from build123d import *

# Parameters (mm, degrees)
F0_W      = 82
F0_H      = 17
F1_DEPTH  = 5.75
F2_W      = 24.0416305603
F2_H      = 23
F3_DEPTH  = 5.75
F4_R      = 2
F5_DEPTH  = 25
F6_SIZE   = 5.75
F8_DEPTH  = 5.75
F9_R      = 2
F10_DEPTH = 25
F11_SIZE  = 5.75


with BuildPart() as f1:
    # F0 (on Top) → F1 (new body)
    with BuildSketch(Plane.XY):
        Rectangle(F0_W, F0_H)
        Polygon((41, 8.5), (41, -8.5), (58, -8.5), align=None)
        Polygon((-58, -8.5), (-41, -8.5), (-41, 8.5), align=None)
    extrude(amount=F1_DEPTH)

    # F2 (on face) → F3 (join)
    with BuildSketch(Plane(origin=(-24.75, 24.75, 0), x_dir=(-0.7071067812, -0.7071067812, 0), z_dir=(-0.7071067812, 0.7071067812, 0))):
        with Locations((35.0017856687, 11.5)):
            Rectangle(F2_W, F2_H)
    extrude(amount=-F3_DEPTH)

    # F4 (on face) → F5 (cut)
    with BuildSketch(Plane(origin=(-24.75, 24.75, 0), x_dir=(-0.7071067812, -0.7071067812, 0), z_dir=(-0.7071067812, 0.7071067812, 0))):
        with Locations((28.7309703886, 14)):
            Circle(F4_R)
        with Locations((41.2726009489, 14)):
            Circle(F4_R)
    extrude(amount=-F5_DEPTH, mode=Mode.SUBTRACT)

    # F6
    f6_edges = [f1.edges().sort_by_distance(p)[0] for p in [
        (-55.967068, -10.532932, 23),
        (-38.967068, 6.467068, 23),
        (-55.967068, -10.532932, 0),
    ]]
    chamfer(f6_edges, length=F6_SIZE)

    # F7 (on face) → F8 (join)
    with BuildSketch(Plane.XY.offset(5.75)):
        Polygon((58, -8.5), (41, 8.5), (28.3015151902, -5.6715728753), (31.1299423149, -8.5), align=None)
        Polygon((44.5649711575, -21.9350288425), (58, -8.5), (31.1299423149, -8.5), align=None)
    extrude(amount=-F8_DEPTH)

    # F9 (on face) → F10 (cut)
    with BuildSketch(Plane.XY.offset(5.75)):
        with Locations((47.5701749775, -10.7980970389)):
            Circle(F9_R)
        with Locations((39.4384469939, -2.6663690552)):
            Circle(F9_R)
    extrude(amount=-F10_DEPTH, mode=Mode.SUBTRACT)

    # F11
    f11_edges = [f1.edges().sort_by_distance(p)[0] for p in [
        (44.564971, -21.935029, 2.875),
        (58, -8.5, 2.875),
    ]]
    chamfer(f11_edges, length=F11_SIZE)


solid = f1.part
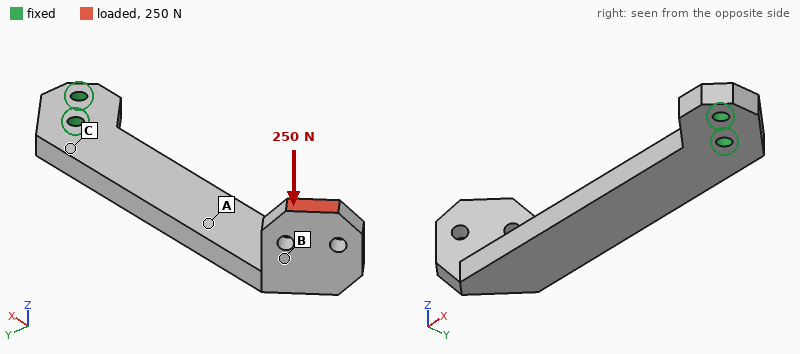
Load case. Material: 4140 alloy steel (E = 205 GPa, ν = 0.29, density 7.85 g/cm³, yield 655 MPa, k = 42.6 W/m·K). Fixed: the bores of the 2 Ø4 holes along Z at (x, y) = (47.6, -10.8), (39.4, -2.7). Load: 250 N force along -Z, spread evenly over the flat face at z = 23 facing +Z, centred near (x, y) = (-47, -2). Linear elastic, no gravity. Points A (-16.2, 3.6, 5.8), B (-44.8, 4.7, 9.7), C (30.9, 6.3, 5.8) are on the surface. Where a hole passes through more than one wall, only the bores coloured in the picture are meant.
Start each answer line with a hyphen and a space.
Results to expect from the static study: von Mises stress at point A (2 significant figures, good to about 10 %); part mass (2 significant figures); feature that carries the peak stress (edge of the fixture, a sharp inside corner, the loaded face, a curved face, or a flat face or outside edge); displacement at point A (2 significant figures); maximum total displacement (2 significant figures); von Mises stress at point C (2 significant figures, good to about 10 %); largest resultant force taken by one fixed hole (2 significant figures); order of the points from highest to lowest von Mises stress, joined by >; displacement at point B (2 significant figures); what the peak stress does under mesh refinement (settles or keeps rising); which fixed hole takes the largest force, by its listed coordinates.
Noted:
- 84 MPa
- 98 g
- edge of the fixture
- 0.47 mm
- 1.2 mm
- 180 MPa
- 700 N
- C > A > B
- 0.94 mm
- keeps rising
- (39.4, -2.7)
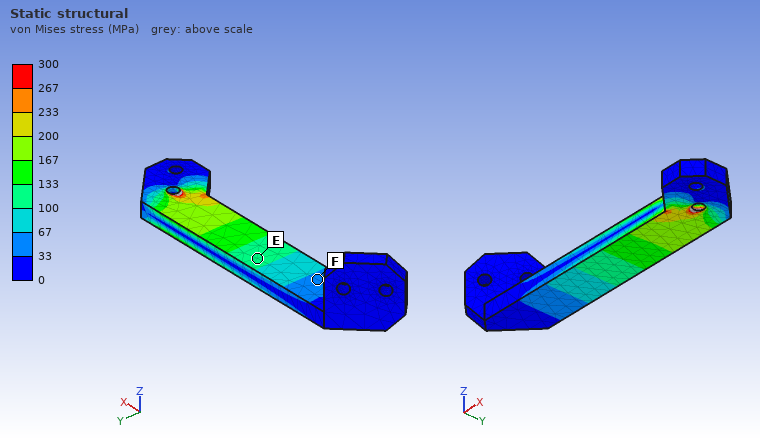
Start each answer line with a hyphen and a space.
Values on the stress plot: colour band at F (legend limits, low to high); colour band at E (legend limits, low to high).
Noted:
- 33 to 67 MPa
- 100 to 133 MPa
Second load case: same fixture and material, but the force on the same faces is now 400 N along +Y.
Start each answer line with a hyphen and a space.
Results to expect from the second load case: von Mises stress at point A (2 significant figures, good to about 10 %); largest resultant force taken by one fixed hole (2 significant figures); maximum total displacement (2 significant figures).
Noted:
- 99 MPa
- 2.2 kN
- 0.44 mm
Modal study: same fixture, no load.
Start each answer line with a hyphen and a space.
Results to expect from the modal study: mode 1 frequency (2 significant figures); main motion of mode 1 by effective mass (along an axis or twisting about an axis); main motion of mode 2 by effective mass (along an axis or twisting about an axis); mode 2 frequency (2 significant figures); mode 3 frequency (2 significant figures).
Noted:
- 430 Hz
- along Z
- along Y
- 1100 Hz
- 2600 Hz
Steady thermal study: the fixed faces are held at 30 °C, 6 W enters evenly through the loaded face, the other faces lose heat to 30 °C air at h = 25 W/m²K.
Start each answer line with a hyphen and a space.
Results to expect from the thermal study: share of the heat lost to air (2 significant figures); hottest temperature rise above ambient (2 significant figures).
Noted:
- 68 %
- 75 K
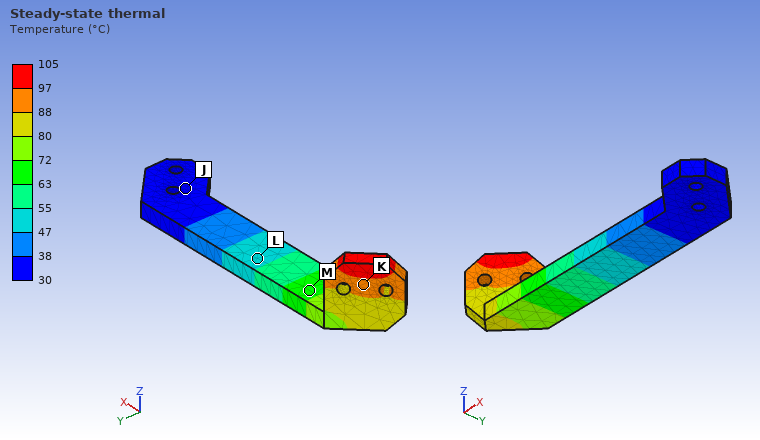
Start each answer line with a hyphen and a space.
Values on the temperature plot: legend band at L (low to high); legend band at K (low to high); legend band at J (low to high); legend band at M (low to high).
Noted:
- 47 to 55 °C
- 88 to 97 °C
- 30 to 38 °C
- 63 to 72 °C
